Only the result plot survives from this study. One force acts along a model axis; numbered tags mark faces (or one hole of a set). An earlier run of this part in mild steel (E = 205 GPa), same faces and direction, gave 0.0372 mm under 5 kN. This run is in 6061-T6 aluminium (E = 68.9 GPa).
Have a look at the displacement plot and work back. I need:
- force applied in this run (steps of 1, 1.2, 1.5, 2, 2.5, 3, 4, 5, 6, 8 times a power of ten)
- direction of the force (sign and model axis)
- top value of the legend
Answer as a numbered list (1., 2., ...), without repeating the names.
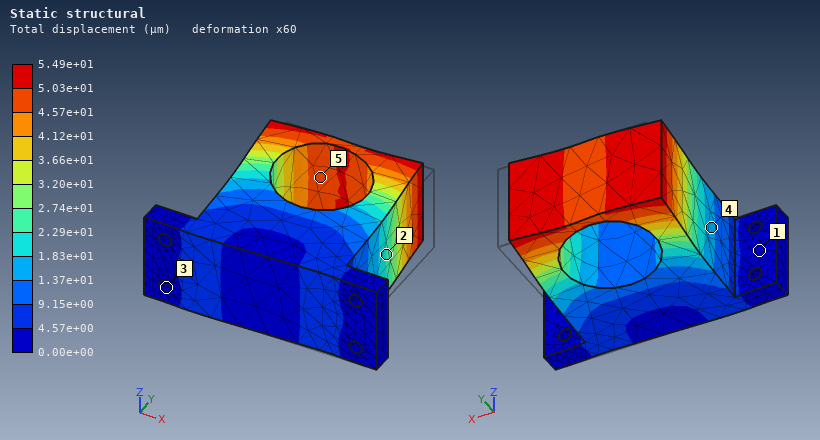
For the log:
1. 2.5 kN
2. -X
3. 5.49e+01 µm
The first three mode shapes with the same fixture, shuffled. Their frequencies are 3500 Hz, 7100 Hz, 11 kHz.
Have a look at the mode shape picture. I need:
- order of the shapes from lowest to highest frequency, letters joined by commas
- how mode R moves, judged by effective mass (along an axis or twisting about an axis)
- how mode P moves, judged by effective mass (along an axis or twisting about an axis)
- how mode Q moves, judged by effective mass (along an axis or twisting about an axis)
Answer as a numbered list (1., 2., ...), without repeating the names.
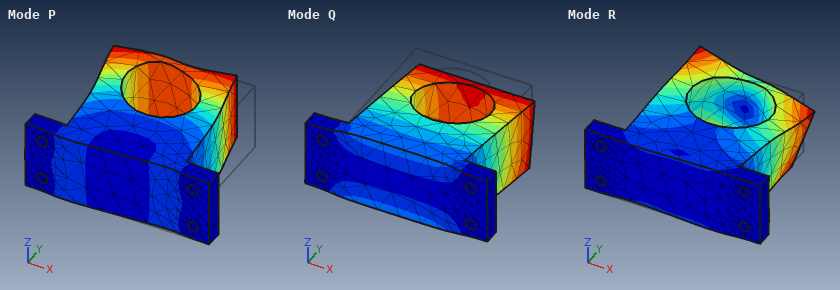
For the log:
1. Q, P, R
2. twisting about Y
3. along X
4. along Z
